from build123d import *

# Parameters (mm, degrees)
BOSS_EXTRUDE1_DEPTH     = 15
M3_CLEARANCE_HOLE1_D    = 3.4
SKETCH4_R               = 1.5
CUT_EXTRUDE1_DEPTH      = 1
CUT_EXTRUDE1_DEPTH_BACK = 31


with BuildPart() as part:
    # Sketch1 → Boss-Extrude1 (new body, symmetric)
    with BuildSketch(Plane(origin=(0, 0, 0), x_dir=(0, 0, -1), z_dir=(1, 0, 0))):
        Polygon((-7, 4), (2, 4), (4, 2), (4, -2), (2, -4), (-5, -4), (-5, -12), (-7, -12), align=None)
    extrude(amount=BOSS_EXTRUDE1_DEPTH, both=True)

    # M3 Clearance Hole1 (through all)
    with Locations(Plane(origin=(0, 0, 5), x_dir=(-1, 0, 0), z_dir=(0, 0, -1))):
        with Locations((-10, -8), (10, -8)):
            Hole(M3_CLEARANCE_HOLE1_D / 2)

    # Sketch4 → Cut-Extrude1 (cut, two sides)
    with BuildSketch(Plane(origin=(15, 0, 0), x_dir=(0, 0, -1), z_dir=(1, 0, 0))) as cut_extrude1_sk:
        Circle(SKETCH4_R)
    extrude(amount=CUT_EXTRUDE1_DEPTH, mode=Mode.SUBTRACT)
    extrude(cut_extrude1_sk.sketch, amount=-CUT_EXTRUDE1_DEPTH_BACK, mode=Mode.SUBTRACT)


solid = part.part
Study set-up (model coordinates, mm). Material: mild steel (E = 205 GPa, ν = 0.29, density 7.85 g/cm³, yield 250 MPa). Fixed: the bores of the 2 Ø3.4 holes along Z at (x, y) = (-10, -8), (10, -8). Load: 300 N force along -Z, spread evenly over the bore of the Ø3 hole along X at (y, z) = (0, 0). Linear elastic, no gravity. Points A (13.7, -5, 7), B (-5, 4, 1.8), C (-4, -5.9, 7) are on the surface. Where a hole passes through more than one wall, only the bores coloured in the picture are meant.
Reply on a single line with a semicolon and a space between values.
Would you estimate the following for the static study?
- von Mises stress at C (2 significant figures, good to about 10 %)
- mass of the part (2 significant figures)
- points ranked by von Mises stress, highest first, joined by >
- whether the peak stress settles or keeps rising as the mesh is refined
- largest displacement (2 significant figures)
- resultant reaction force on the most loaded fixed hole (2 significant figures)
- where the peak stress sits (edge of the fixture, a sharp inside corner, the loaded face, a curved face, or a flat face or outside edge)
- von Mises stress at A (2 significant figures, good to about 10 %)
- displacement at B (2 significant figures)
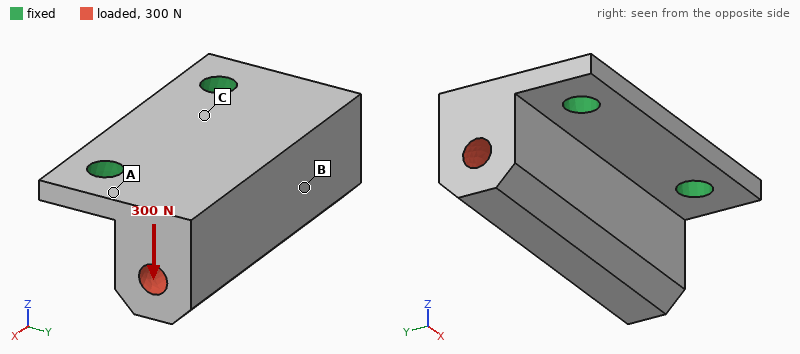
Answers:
43 MPa; 22 g; A > C > B; keeps rising; 23 µm; 150 N; edge of the fixture; 66 MPa; 19 µm
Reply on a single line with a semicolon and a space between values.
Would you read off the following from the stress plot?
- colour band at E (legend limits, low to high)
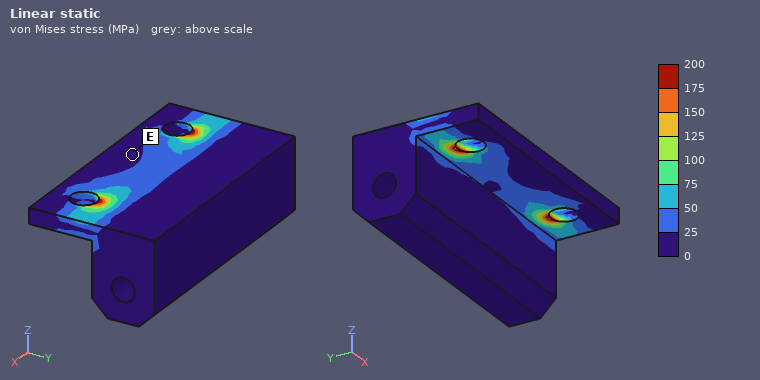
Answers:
0 to 25 MPa
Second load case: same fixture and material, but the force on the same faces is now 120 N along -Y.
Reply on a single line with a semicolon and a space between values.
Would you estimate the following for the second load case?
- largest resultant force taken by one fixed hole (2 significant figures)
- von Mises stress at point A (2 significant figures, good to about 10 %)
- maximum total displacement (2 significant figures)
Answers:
61 N; 31 MPa; 10 µm
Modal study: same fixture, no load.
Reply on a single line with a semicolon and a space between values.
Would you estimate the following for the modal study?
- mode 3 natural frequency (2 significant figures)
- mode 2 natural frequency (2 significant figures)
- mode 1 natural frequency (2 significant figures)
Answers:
24 kHz; 16 kHz; 4500 Hz
